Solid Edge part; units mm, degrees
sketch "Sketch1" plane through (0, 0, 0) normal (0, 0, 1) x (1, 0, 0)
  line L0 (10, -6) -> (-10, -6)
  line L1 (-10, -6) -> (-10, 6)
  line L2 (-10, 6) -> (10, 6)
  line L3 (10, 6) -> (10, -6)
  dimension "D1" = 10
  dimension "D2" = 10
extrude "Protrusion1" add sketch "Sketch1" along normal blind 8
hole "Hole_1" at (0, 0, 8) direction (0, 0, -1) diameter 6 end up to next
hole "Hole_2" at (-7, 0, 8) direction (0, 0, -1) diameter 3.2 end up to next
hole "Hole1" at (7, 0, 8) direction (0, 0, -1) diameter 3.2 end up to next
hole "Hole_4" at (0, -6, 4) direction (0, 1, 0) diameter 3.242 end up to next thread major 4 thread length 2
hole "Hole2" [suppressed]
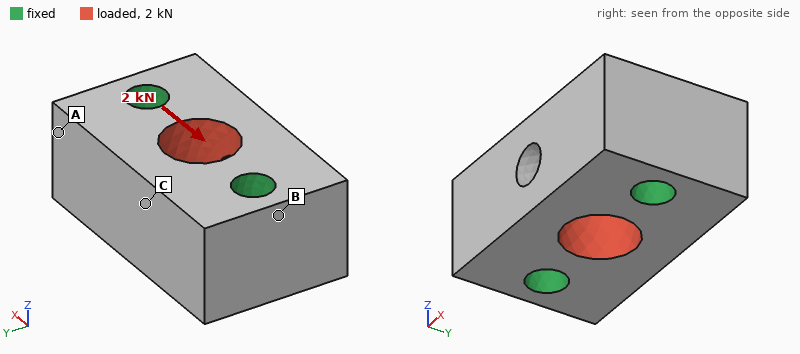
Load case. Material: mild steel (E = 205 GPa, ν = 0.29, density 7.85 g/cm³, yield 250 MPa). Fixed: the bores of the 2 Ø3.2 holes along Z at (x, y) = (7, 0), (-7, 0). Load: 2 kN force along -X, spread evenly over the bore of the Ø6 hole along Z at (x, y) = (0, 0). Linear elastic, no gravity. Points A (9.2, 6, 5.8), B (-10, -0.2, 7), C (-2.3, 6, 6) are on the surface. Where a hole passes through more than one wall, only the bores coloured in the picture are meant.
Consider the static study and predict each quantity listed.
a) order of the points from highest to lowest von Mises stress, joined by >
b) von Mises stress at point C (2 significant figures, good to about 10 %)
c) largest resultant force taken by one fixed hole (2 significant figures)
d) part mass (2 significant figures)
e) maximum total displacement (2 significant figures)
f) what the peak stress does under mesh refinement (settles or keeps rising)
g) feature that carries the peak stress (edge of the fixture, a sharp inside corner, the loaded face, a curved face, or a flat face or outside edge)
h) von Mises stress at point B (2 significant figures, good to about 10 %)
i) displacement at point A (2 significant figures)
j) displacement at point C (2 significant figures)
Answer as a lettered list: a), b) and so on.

a) B > C > A
b) 5.1 MPa
c) 1.0 kN
d) 12 g
e) 0.60 µm
f) keeps rising
g) edge of the fixture
h) 9.4 MPa
i) 0.37 µm
j) 0.35 µm
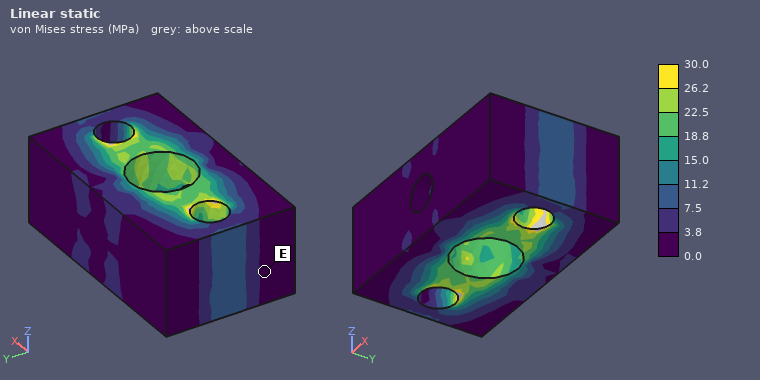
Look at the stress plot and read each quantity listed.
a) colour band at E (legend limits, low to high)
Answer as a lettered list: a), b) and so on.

a) 0.0 to 3.8 MPa
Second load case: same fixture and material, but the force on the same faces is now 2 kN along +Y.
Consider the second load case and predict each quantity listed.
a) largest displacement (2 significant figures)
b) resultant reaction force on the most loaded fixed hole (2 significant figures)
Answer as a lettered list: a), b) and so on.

a) 1.2 µm
b) 1.0 kN
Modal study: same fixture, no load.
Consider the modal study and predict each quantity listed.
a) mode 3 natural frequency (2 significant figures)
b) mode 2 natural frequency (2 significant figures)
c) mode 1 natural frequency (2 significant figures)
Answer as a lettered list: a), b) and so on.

a) 97 kHz
b) 94 kHz
c) 89 kHz
